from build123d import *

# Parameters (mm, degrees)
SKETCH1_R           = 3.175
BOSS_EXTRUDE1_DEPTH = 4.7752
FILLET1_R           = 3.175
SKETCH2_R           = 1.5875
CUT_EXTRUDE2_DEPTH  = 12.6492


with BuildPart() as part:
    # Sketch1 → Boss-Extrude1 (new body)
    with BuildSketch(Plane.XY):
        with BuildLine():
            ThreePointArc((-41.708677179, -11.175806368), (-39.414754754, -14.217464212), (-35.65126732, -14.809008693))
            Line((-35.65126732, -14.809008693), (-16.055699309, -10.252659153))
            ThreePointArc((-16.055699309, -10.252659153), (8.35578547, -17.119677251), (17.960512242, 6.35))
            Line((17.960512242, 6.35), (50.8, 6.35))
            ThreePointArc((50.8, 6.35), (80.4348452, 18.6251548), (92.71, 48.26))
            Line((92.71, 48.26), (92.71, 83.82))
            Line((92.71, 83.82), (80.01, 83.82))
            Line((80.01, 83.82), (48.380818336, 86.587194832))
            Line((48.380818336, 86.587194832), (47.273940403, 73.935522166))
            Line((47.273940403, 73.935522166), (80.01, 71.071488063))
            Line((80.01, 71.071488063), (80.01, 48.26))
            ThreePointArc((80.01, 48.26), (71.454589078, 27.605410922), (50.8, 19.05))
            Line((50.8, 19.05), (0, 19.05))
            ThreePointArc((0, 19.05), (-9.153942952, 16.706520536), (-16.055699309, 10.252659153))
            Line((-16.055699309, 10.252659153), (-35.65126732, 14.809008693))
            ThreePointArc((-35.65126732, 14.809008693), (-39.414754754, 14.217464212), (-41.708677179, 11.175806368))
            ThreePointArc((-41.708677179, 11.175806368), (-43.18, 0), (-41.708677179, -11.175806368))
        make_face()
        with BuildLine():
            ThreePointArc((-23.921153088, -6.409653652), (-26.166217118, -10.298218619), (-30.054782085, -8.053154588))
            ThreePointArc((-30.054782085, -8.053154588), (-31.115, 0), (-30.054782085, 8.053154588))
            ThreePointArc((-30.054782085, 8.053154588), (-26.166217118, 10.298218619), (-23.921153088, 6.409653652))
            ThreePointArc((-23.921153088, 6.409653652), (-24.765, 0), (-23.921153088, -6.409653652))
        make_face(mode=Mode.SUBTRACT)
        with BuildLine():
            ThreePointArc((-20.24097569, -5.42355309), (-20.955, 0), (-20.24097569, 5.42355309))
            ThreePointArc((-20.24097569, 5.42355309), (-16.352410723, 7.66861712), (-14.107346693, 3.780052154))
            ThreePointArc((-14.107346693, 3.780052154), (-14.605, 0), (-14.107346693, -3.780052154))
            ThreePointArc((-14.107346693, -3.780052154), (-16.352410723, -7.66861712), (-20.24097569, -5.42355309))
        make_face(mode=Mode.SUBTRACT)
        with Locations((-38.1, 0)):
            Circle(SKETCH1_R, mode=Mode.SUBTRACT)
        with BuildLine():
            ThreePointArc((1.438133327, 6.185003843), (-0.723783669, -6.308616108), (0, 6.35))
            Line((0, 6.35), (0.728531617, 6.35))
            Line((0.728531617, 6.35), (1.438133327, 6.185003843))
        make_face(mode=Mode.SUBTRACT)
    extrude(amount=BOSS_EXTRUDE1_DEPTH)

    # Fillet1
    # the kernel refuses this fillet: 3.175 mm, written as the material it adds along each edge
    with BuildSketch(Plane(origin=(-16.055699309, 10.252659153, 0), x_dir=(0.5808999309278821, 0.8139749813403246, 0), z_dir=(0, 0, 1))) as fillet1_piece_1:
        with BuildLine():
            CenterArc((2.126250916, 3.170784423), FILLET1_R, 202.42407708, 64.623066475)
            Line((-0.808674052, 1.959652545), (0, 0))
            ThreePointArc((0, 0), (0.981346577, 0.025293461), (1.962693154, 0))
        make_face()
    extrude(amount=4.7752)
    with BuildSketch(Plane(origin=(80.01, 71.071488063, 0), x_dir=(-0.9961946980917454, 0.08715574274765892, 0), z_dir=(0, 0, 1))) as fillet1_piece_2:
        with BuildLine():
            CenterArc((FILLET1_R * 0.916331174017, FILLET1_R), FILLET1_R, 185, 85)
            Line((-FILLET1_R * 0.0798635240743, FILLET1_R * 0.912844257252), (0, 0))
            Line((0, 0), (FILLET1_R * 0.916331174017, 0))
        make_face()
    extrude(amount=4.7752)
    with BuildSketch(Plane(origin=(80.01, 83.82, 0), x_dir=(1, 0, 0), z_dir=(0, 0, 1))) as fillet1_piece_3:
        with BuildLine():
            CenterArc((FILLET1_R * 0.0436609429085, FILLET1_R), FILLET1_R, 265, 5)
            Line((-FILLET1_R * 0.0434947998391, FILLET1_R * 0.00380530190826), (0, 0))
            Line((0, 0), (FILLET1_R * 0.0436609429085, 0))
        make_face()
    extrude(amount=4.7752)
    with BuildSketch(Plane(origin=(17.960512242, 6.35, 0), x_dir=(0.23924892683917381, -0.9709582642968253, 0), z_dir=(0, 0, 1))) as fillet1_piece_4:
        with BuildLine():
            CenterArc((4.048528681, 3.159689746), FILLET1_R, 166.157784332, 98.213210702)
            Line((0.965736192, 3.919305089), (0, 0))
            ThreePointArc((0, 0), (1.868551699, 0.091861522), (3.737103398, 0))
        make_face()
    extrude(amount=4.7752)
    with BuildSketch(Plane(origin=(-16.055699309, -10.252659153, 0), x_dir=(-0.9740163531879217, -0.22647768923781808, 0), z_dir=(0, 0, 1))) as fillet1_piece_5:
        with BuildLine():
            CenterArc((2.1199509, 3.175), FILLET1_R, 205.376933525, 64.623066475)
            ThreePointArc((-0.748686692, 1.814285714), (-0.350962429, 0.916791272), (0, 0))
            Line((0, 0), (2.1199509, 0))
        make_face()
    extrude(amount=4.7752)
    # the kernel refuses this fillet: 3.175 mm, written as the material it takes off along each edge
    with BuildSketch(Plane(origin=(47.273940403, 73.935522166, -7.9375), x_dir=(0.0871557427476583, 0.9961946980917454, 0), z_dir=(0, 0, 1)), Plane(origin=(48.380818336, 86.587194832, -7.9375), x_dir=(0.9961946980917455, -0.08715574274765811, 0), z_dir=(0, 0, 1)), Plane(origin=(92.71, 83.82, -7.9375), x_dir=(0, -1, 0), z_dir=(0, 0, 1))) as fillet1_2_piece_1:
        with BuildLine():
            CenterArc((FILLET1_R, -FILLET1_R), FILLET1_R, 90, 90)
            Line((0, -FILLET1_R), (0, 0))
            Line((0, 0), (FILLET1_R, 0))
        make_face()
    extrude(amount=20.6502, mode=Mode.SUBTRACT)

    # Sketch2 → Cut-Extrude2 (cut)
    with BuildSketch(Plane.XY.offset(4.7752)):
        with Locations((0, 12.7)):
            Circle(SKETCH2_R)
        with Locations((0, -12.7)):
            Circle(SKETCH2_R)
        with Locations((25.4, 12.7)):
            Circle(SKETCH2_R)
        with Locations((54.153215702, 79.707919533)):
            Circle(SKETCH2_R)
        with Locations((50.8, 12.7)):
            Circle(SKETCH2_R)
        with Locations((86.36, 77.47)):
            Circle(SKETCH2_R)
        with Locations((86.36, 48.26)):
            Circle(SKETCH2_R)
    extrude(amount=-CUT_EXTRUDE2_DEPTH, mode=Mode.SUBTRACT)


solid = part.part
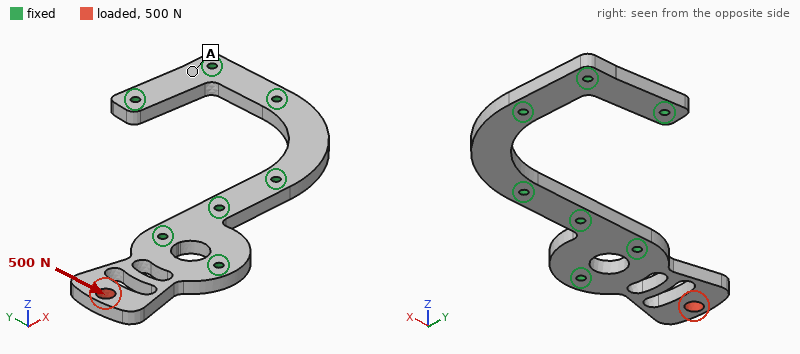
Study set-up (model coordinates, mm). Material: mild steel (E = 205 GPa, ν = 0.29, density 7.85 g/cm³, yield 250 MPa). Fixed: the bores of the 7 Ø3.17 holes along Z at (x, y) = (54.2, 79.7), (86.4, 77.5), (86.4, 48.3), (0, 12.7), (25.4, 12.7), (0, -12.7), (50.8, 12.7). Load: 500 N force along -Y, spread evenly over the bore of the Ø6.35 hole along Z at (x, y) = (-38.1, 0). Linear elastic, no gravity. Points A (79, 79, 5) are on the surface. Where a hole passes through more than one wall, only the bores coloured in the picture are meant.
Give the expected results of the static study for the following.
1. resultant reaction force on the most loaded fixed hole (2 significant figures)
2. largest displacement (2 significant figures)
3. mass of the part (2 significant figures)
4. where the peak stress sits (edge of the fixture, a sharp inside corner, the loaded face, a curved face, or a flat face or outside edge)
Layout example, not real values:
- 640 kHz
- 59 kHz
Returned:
- 730 N
- 34 µm
- 130 g
- a curved face
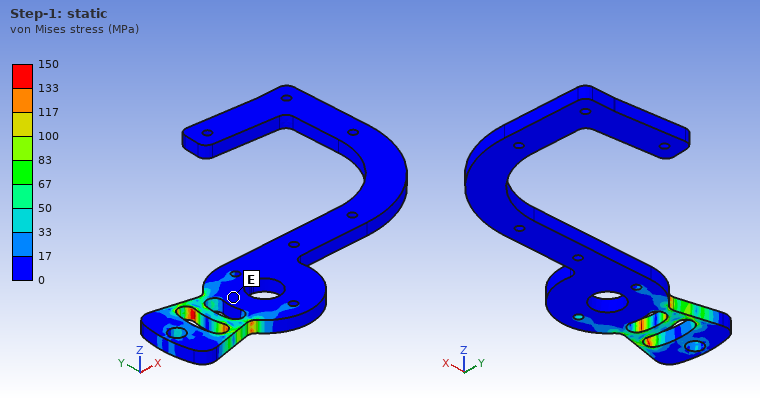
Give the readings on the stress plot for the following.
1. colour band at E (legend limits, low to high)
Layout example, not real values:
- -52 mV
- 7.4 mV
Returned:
- 0 to 17 MPa
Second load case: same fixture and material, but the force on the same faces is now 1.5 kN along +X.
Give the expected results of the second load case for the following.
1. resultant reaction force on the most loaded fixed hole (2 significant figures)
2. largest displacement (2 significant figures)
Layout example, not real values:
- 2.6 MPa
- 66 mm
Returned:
- 760 N
- 13 µm
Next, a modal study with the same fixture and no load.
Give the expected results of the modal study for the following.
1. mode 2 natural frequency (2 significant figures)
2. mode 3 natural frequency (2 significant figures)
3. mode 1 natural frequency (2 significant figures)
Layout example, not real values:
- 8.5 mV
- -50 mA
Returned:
- 5300 Hz
- 5900 Hz
- 1800 Hz
